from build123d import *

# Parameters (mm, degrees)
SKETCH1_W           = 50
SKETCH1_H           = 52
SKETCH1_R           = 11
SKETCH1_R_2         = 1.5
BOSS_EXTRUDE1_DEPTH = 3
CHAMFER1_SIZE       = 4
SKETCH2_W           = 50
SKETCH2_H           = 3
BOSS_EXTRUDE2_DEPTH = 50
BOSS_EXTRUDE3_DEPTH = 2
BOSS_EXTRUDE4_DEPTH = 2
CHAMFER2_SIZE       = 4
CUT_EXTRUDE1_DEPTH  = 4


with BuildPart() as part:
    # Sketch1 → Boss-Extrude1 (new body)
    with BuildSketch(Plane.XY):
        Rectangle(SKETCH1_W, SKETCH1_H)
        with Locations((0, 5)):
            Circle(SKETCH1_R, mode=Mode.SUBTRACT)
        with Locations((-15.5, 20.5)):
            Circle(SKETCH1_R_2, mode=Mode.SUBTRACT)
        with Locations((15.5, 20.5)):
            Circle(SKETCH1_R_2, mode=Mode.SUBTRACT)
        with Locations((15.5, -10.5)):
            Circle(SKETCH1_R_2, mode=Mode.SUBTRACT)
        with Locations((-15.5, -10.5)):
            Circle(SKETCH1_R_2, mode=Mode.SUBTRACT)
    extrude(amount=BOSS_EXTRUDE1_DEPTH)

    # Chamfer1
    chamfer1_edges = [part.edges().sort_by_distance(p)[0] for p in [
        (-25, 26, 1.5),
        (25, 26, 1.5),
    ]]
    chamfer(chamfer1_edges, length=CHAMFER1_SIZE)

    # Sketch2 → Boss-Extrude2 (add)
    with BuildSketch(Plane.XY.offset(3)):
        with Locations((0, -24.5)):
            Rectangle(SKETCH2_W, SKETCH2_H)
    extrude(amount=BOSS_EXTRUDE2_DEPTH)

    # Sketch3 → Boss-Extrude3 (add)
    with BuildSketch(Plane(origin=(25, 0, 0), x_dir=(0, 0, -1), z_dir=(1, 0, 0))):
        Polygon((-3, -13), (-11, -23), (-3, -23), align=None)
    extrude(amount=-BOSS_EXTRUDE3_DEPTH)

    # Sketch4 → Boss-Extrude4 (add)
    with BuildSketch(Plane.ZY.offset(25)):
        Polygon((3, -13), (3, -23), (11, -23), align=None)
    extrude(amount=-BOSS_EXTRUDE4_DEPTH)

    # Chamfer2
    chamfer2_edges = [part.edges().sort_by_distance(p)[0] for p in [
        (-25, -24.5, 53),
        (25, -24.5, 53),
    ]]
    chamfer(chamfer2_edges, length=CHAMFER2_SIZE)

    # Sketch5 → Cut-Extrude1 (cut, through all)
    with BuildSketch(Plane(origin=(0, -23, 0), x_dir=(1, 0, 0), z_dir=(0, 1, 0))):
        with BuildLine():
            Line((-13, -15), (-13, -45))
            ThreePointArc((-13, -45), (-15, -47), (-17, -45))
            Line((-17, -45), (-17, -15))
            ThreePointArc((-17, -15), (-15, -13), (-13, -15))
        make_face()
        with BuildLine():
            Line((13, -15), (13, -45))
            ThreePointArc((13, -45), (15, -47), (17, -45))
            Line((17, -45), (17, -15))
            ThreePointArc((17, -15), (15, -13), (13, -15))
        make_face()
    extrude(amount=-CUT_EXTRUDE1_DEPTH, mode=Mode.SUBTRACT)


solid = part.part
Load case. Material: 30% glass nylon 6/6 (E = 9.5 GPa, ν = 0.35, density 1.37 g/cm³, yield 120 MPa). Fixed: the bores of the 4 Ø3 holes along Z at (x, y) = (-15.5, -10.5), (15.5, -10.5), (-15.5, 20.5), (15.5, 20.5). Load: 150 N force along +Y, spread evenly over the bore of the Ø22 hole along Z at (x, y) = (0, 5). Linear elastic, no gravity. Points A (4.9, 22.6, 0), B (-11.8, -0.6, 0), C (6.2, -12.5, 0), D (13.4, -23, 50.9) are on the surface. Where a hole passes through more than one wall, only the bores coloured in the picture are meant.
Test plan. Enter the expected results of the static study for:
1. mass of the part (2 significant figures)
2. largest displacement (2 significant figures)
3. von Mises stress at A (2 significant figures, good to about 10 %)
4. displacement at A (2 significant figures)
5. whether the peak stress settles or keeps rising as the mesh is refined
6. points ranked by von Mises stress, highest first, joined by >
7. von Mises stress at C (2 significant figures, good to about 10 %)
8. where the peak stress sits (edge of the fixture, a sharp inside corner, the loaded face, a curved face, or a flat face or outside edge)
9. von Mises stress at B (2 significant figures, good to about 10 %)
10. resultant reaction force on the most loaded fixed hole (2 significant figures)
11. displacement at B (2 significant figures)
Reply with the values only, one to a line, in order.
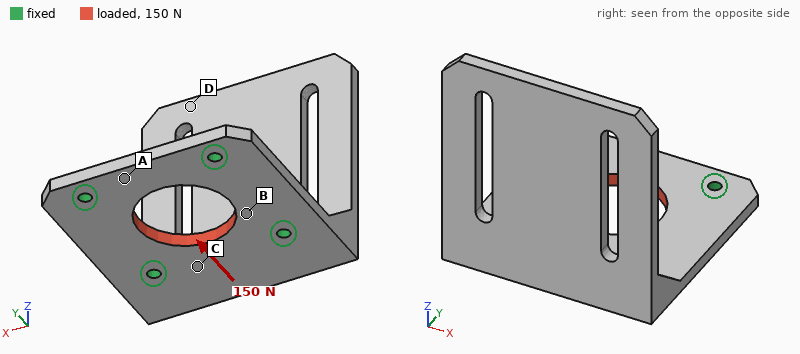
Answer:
18 g
3.5 µm
0.74 MPa
2.7 µm
keeps rising
B > A > C > D
0.53 MPa
edge of the fixture
1.1 MPa
39 N
1.1 µm
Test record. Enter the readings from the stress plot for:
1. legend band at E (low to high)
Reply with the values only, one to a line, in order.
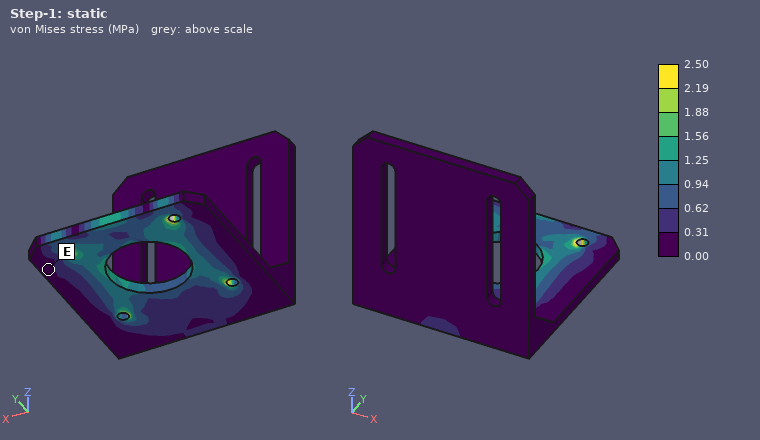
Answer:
0.00 to 0.31 MPa
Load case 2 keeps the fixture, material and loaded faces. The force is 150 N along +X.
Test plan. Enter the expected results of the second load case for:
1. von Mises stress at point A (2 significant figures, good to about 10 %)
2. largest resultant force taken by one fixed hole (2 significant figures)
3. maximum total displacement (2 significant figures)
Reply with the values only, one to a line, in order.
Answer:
0.53 MPa
39 N
2.6 µm
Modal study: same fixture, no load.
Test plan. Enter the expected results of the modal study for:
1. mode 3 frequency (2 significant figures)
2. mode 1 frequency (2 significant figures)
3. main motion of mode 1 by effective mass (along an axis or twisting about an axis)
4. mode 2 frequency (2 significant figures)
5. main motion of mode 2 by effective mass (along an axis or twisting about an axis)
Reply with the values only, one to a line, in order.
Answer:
1400 Hz
390 Hz
along Y
940 Hz
along X
